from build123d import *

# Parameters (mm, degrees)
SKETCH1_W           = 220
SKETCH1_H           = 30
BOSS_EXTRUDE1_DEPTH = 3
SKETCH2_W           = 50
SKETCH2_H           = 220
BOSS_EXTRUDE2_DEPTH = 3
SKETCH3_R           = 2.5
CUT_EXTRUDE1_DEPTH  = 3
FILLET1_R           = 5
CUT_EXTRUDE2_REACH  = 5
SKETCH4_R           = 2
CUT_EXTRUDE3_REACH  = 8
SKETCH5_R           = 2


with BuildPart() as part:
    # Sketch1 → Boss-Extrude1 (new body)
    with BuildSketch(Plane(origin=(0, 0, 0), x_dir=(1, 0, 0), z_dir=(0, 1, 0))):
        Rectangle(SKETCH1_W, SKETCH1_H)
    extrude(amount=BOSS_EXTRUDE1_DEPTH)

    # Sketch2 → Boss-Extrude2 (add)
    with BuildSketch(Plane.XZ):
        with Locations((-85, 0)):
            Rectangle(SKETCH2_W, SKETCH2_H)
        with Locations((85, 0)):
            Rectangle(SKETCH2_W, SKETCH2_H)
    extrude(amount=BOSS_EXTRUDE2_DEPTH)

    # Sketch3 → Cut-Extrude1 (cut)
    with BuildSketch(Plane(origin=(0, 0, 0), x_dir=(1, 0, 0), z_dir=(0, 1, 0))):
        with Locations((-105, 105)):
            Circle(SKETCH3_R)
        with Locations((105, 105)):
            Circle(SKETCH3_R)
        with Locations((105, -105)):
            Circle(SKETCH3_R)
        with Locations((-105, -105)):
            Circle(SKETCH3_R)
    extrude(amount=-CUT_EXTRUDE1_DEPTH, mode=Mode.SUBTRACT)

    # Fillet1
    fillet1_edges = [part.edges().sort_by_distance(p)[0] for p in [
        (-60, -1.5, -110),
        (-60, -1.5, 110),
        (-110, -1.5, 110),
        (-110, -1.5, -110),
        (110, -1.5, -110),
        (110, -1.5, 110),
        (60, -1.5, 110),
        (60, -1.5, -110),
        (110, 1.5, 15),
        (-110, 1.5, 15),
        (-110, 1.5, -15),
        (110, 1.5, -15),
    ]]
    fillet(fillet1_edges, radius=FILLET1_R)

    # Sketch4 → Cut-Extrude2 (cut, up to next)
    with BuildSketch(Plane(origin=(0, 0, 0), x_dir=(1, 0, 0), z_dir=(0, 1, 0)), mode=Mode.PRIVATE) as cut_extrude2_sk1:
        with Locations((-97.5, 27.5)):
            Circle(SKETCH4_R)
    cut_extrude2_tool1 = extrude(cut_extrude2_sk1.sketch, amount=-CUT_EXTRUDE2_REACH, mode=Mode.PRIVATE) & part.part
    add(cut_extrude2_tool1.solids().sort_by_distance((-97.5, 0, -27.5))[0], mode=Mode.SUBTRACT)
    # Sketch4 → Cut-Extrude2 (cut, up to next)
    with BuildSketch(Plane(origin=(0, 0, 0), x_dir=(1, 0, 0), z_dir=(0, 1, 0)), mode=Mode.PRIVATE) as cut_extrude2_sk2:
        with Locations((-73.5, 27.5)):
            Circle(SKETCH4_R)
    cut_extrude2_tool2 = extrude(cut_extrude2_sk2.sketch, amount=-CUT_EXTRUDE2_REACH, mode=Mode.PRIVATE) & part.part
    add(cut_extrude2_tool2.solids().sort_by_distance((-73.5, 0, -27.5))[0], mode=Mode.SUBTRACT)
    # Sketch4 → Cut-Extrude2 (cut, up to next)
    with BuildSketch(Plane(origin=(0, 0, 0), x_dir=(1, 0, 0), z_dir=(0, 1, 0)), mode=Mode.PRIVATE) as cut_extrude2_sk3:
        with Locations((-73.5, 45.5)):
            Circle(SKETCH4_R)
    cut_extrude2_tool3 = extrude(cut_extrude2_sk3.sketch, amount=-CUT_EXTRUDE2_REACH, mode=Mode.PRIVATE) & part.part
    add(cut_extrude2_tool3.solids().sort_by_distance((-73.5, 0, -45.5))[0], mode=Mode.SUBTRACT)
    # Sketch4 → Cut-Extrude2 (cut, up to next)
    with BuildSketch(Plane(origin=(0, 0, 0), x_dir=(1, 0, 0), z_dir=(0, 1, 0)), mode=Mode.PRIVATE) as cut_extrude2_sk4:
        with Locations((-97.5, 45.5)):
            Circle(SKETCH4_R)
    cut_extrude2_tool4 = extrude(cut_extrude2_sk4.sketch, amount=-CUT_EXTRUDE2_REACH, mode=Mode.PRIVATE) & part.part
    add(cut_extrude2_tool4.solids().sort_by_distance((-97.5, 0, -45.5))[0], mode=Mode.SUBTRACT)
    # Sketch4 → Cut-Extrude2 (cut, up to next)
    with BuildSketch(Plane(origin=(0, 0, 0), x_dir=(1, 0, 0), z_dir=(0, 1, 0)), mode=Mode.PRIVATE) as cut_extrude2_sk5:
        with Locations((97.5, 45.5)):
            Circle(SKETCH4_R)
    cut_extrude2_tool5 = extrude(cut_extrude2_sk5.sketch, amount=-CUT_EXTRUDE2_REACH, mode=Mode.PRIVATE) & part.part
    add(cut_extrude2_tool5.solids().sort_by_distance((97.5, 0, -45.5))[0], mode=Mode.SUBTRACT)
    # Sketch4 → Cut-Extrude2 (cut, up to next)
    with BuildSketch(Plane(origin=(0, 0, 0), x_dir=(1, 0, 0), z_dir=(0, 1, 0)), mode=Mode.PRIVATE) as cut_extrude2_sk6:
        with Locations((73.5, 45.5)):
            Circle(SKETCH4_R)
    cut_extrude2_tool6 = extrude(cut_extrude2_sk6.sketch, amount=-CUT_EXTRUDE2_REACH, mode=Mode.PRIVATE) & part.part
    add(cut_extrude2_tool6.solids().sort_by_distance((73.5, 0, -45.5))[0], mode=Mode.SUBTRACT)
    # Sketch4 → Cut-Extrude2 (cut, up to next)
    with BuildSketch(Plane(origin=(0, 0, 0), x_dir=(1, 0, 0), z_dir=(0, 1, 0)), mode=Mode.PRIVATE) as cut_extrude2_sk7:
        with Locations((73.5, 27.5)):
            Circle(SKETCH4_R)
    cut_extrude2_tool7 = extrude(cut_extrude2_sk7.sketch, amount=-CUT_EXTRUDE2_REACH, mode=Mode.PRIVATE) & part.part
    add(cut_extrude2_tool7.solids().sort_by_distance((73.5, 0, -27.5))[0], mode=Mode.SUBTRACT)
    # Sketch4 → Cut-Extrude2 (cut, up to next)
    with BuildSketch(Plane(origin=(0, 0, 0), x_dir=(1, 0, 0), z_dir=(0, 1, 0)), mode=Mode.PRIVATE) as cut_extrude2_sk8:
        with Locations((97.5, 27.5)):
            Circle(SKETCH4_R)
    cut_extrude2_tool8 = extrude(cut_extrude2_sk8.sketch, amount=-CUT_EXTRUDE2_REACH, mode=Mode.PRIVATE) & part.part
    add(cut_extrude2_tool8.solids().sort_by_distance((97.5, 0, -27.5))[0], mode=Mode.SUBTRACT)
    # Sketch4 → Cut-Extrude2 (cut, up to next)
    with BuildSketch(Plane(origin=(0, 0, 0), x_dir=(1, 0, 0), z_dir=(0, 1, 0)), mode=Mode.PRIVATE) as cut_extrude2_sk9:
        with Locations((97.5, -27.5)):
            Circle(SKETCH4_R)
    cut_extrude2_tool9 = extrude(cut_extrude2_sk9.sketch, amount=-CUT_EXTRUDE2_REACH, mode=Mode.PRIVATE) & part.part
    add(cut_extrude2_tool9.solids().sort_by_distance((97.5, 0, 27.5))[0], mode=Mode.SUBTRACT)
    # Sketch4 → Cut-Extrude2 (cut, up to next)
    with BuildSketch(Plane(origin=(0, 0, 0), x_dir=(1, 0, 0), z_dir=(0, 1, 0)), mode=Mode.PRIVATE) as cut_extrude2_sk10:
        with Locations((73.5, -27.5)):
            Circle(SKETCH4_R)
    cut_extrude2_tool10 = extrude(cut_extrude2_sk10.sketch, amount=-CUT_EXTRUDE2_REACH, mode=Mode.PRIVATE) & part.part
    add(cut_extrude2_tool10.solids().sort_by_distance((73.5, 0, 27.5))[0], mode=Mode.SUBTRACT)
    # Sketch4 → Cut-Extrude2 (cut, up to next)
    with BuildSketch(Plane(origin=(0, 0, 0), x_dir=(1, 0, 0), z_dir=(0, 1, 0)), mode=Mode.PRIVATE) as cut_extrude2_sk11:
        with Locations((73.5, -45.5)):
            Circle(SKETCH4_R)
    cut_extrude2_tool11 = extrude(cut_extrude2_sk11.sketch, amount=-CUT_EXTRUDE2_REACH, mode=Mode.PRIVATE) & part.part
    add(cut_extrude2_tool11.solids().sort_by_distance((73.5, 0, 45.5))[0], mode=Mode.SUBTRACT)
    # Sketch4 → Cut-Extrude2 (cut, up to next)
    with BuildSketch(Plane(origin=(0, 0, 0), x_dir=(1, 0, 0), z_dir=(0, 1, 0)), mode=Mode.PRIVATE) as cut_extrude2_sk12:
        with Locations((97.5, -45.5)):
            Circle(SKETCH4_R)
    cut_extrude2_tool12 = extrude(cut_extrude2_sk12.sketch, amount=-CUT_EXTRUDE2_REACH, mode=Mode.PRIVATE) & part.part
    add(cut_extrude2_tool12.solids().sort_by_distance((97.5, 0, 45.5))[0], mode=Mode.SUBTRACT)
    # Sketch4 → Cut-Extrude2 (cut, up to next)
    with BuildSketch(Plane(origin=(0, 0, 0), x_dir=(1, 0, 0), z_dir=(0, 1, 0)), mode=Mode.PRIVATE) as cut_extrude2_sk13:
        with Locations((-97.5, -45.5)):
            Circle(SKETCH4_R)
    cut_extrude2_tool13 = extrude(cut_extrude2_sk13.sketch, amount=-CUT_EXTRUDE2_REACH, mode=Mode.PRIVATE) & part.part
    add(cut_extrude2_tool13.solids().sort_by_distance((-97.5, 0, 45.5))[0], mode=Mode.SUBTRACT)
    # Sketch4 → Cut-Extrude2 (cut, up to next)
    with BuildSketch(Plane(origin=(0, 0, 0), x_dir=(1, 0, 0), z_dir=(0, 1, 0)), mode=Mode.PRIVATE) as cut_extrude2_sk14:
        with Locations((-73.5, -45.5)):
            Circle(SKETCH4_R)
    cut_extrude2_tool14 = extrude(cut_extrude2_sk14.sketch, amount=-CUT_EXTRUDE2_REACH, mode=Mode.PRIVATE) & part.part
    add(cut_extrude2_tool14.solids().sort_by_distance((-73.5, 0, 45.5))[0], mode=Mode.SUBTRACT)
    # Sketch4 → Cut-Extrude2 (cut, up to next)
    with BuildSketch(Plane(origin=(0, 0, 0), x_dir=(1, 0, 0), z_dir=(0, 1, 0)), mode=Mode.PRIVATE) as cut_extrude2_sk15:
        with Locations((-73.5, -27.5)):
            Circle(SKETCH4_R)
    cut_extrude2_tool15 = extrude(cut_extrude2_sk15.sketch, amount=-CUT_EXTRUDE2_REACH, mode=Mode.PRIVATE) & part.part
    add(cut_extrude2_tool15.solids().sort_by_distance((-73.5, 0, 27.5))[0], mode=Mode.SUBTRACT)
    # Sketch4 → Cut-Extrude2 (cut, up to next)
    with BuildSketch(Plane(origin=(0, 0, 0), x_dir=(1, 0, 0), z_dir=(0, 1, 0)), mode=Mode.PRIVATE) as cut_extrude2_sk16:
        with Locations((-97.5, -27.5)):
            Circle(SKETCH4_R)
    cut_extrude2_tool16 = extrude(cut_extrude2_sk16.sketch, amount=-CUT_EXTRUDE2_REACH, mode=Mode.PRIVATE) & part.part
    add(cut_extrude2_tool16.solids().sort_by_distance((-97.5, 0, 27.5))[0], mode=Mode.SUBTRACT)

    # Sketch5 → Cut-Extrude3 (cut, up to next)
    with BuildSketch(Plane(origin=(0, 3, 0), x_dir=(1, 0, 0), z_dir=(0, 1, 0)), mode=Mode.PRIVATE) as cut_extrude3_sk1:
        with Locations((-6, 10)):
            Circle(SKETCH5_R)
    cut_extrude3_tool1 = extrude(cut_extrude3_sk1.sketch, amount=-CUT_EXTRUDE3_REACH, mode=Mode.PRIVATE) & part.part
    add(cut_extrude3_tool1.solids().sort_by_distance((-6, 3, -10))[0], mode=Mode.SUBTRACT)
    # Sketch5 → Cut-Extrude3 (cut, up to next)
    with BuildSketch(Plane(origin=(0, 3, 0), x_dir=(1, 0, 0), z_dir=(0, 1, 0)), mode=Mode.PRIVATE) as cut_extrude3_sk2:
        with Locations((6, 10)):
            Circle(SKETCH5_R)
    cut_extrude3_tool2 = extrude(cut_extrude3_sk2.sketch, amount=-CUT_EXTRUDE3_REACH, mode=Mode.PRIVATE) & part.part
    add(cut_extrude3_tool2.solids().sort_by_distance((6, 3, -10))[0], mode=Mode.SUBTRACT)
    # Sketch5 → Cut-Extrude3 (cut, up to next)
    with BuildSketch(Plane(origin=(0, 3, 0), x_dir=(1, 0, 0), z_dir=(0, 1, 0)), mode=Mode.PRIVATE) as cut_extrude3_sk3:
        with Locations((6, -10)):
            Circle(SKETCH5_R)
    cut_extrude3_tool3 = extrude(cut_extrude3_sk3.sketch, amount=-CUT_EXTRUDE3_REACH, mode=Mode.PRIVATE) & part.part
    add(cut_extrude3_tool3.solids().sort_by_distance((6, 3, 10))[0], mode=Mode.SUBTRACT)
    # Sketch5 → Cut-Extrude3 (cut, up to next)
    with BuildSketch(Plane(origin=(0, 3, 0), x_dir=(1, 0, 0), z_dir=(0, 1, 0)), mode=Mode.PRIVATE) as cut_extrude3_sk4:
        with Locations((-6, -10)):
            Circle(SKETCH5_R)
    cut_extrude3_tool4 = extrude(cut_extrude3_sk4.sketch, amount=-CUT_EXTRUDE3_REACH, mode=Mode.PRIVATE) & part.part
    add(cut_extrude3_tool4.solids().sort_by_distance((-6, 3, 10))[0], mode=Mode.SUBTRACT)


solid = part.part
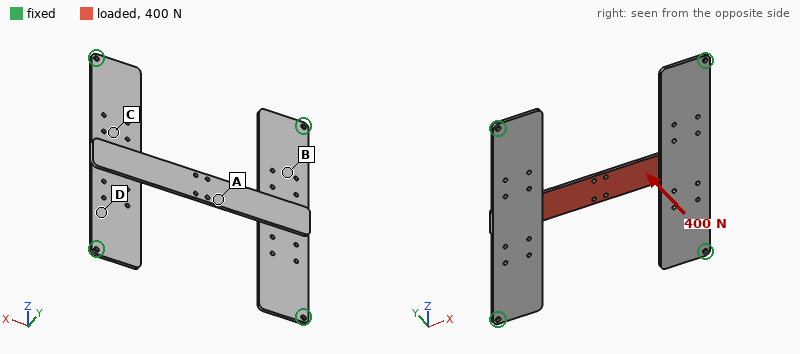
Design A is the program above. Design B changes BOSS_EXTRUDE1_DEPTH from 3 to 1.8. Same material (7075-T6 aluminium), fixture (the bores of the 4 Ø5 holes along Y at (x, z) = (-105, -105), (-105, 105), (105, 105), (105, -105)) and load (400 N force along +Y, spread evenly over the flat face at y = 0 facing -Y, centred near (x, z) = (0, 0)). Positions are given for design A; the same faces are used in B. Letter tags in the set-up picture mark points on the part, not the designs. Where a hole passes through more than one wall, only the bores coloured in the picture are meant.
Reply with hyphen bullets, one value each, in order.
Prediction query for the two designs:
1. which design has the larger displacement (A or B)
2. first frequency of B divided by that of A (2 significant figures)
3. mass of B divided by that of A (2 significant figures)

- B
- 1.1
- 0.91
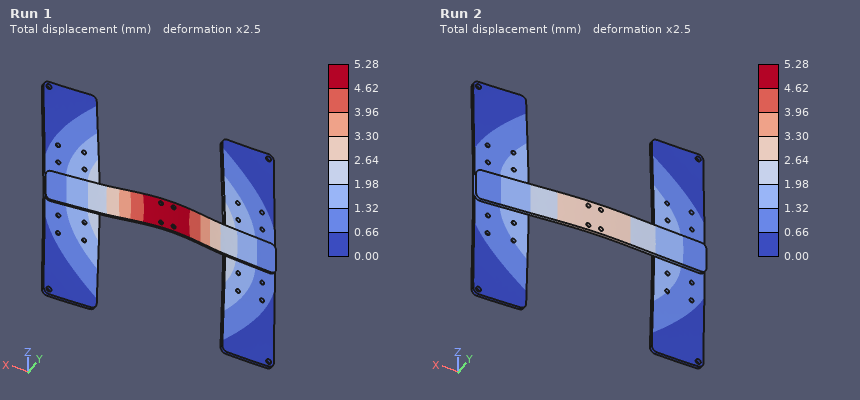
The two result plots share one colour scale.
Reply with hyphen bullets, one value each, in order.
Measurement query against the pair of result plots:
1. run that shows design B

- Run 1
